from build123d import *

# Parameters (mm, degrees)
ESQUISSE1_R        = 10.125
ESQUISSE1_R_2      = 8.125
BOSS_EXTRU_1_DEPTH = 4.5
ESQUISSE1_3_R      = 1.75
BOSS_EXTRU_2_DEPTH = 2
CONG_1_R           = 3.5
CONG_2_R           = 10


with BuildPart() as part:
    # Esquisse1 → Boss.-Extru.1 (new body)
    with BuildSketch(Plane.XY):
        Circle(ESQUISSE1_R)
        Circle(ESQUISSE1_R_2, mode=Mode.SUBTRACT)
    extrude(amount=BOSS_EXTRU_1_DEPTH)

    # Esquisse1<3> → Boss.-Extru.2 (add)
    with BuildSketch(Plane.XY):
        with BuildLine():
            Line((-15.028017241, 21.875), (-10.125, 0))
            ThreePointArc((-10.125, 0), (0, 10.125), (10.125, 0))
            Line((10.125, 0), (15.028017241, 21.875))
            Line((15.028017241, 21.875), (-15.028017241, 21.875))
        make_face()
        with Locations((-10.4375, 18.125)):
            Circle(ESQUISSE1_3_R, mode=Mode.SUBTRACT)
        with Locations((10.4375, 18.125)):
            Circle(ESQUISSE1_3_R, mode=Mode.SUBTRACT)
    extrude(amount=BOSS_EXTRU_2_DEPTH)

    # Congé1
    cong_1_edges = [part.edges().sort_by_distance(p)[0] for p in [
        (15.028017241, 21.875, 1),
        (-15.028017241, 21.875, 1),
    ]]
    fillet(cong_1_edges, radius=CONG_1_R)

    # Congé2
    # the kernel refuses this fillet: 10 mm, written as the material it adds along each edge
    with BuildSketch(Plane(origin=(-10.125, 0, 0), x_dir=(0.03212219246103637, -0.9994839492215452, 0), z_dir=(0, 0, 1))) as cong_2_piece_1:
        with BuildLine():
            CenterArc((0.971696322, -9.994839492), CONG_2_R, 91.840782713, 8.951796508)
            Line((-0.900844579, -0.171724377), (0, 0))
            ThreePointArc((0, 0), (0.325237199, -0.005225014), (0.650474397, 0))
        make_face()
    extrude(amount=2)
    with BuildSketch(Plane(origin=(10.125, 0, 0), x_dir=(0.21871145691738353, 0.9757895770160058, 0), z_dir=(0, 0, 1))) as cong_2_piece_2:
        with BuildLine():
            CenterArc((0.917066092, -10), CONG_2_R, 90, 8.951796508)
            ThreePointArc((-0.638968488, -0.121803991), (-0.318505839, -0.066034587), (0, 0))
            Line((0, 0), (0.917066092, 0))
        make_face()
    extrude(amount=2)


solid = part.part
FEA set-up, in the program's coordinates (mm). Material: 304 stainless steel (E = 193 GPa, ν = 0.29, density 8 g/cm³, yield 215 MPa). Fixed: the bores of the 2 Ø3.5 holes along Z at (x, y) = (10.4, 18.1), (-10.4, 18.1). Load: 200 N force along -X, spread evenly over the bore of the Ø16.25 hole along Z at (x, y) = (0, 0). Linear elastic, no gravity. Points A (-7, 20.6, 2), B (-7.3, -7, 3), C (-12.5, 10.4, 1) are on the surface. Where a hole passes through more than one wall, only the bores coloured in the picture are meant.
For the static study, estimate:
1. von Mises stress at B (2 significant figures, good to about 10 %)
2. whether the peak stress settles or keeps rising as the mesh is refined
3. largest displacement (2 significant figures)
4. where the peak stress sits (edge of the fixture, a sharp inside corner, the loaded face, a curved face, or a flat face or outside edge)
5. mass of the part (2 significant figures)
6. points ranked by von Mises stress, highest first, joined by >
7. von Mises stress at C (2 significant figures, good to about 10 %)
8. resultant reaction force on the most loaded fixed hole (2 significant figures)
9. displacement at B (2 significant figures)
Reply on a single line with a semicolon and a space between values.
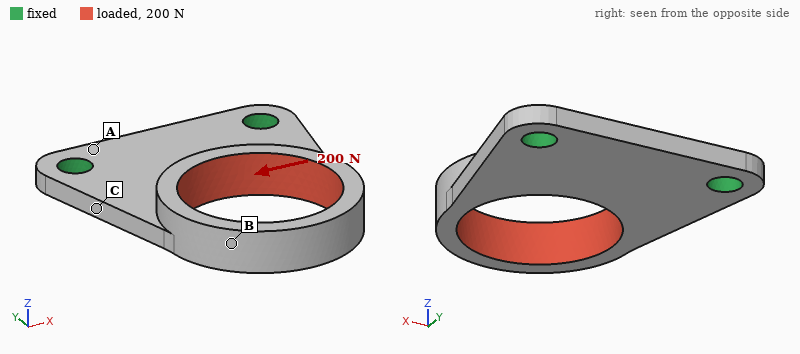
32 MPa; keeps rising; 13 µm; a sharp inside corner; 9.9 g; B > C > A; 21 MPa; 190 N; 13 µm
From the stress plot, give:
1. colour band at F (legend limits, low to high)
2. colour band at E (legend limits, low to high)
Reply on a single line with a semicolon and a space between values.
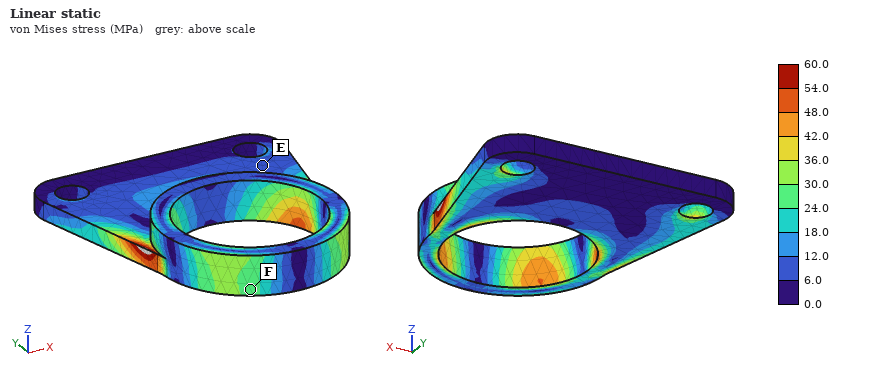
24.0 to 30.0 MPa; 6.0 to 12.0 MPa
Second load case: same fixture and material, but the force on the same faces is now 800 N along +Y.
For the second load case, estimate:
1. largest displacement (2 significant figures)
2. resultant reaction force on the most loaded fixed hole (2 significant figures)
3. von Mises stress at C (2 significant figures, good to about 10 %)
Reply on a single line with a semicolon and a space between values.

92 µm; 410 N; 36 MPa
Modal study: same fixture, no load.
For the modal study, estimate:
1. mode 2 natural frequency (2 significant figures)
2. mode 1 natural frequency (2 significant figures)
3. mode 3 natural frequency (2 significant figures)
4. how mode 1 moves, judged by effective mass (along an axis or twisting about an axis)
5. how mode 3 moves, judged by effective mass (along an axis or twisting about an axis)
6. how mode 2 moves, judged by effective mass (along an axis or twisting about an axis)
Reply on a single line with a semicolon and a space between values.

8200 Hz; 2700 Hz; 11 kHz; along Z; along X; twisting about Y
